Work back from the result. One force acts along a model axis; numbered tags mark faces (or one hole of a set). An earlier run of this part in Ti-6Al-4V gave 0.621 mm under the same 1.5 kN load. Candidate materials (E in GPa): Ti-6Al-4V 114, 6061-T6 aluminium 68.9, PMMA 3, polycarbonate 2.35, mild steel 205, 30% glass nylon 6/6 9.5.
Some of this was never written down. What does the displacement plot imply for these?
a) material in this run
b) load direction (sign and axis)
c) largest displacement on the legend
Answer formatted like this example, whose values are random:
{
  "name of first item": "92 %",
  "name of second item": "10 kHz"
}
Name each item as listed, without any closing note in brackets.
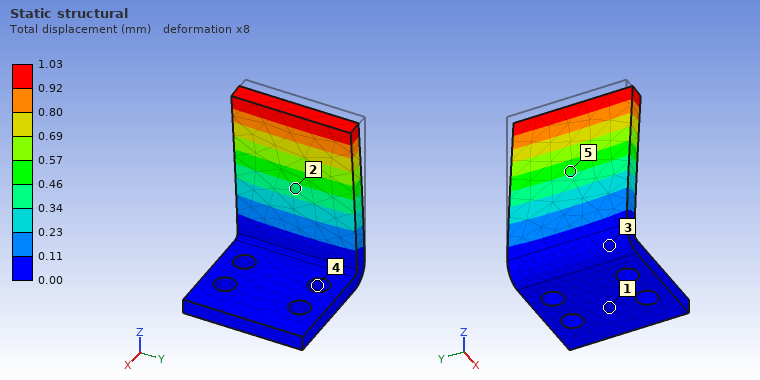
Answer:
{
  "material in this run": "6061-T6 aluminium",
  "load direction": "+X",
  "largest displacement on the legend": "1.03 mm"
}
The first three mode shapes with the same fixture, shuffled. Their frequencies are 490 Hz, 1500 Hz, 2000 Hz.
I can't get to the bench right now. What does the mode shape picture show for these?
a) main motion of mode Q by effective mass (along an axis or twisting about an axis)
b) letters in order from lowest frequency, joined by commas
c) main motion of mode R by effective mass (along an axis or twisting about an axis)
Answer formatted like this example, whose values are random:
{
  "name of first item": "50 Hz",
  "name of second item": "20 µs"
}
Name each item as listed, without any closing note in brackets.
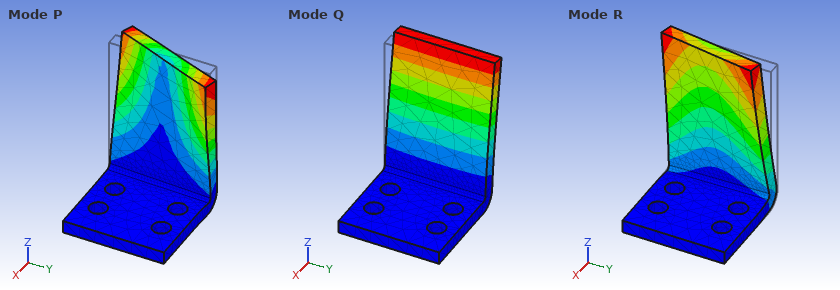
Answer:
{
  "main motion of mode Q by effective mass": "along X",
  "letters in order from lowest frequency, joined by commas": "Q, R, P",
  "main motion of mode R by effective mass": "along Y"
}
